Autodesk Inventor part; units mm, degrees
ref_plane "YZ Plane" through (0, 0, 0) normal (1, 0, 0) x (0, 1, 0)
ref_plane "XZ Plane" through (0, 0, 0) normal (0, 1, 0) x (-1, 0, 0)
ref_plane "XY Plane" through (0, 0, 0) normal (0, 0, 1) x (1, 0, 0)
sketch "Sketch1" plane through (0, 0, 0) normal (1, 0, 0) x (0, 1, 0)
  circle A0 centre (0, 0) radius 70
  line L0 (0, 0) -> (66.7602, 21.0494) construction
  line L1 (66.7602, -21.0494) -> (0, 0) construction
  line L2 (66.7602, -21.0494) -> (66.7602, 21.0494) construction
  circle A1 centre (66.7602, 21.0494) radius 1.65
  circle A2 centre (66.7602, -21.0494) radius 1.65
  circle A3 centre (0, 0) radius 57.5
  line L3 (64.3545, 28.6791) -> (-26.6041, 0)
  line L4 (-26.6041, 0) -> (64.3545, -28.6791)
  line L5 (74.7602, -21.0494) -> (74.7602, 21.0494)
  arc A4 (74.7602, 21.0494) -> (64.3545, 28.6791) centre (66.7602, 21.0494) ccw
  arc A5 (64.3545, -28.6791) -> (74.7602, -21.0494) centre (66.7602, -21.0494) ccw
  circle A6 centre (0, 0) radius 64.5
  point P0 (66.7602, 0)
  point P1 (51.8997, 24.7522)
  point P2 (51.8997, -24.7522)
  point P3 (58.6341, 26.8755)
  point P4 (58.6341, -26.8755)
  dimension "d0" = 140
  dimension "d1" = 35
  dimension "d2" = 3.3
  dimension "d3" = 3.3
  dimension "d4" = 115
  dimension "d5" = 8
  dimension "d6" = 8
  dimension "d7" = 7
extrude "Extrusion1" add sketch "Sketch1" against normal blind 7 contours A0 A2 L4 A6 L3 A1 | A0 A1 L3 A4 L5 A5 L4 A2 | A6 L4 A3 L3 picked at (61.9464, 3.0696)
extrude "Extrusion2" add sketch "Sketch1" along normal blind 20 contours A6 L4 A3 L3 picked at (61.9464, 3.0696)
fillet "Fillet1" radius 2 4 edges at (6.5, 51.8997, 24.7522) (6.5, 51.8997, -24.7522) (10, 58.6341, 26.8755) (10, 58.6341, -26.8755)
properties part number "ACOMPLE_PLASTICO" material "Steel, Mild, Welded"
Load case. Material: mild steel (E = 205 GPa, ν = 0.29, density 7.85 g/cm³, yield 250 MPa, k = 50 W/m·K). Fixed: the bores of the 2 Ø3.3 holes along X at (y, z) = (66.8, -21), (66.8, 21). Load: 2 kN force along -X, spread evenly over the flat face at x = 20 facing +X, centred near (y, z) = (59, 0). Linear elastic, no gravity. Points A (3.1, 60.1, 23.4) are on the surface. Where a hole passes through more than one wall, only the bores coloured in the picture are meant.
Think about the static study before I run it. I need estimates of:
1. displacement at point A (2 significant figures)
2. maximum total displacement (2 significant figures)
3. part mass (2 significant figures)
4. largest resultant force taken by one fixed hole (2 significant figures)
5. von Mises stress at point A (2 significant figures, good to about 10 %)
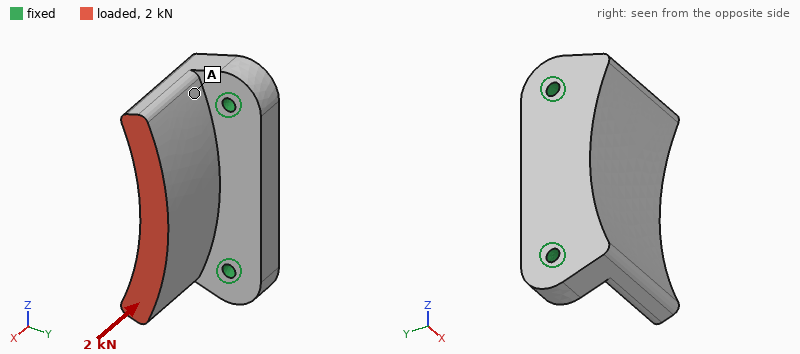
3.9 µm
11 µm
110 g
1.0 kN
16 MPa
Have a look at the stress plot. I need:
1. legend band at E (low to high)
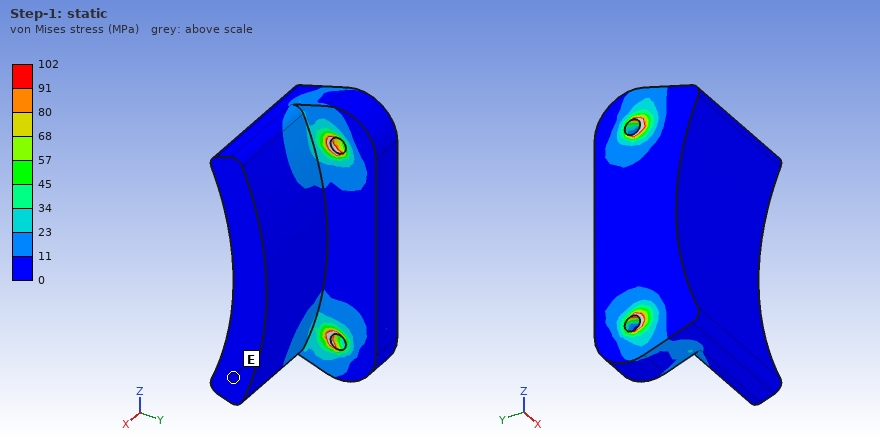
0 to 11 MPa
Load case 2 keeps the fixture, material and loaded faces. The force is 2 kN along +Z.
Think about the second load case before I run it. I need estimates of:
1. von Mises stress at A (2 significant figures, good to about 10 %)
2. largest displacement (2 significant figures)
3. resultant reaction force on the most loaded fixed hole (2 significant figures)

29 MPa
7.9 µm
1.5 kN
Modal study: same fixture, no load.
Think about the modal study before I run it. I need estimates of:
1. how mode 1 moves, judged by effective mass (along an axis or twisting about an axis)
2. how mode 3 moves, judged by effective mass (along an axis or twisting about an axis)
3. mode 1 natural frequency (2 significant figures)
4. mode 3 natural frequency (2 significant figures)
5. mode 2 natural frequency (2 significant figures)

along Y
along X
5900 Hz
15 kHz
11 kHz
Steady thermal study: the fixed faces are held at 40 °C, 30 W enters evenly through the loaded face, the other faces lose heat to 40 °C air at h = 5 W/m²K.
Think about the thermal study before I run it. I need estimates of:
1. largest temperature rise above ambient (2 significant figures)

56 K
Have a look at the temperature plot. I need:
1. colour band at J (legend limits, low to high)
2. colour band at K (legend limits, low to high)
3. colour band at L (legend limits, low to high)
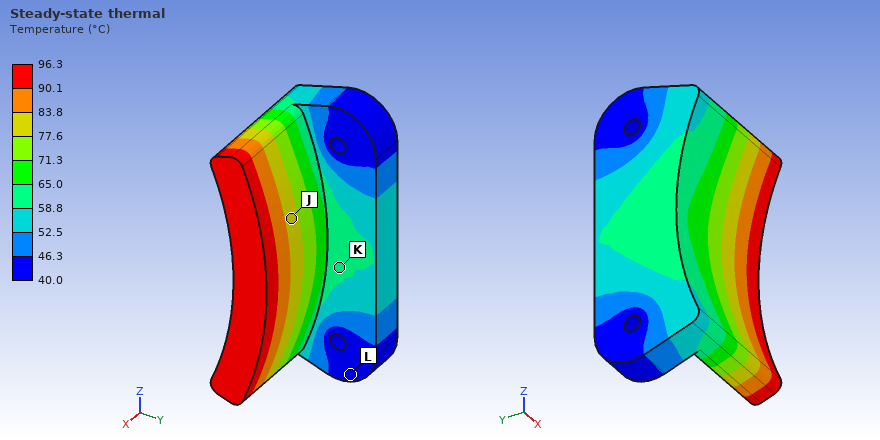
77.6 to 83.8 °C
58.8 to 65.0 °C
40.0 to 46.3 °C
